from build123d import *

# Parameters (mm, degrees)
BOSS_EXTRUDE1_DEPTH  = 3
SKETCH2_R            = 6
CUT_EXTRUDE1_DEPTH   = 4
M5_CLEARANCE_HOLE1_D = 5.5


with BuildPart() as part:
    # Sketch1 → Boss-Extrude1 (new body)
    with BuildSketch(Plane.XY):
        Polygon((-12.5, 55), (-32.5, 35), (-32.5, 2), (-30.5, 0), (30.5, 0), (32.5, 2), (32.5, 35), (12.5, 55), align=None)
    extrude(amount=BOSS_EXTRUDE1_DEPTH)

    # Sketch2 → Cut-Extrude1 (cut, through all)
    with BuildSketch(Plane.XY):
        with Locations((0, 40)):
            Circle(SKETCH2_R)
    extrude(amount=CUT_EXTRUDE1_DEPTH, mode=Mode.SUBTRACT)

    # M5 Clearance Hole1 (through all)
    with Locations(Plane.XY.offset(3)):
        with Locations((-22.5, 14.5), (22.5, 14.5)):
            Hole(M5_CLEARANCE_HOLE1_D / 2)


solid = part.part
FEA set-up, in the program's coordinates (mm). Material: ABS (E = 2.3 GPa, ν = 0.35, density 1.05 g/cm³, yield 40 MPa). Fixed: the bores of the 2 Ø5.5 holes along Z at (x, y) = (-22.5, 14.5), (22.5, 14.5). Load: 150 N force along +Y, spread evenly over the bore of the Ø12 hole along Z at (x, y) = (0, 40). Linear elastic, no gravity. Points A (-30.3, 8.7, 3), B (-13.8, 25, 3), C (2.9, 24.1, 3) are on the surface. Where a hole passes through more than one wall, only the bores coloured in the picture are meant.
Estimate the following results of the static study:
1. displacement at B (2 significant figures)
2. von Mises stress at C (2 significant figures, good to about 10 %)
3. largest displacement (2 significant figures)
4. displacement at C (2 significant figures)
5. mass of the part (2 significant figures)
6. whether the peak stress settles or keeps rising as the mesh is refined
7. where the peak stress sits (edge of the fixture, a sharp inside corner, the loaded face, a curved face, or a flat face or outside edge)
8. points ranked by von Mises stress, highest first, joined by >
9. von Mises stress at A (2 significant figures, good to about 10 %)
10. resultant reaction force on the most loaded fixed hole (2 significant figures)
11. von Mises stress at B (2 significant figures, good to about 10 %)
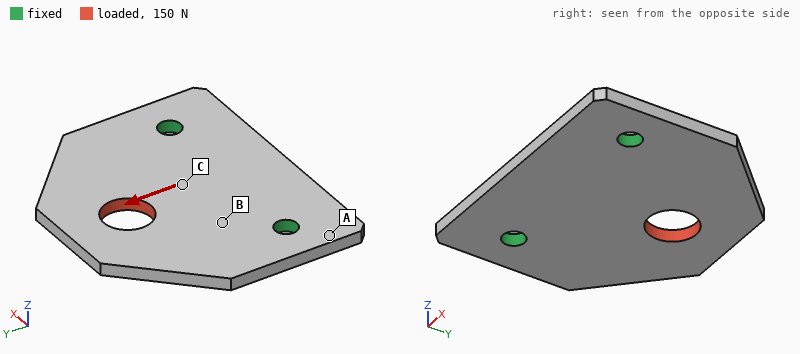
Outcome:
9.6 µm
0.84 MPa
30 µm
14 µm
9.5 g
keeps rising
edge of the fixture
B > C > A
0.37 MPa
78 N
1.4 MPa
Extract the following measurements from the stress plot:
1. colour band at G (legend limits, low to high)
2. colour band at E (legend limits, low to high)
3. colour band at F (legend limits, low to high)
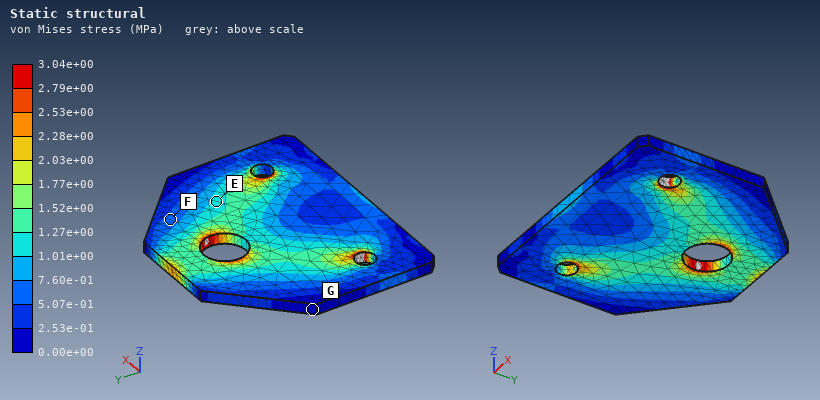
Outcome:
0.00e+00 to 2.53e-01 MPa
1.01e+00 to 1.27e+00 MPa
5.07e-01 to 7.60e-01 MPa
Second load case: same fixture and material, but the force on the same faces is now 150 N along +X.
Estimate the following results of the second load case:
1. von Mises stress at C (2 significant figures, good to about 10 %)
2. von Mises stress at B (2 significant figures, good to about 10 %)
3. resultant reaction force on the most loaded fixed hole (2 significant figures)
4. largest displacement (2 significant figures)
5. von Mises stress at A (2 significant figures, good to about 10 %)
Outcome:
1.9 MPa
1.7 MPa
110 N
52 µm
0.78 MPa
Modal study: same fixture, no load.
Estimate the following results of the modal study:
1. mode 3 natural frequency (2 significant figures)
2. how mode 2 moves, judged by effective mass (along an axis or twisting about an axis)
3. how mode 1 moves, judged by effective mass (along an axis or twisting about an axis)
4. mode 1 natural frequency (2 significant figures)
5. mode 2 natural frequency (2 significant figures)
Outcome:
2100 Hz
twisting about Y
along Z
530 Hz
1200 Hz
